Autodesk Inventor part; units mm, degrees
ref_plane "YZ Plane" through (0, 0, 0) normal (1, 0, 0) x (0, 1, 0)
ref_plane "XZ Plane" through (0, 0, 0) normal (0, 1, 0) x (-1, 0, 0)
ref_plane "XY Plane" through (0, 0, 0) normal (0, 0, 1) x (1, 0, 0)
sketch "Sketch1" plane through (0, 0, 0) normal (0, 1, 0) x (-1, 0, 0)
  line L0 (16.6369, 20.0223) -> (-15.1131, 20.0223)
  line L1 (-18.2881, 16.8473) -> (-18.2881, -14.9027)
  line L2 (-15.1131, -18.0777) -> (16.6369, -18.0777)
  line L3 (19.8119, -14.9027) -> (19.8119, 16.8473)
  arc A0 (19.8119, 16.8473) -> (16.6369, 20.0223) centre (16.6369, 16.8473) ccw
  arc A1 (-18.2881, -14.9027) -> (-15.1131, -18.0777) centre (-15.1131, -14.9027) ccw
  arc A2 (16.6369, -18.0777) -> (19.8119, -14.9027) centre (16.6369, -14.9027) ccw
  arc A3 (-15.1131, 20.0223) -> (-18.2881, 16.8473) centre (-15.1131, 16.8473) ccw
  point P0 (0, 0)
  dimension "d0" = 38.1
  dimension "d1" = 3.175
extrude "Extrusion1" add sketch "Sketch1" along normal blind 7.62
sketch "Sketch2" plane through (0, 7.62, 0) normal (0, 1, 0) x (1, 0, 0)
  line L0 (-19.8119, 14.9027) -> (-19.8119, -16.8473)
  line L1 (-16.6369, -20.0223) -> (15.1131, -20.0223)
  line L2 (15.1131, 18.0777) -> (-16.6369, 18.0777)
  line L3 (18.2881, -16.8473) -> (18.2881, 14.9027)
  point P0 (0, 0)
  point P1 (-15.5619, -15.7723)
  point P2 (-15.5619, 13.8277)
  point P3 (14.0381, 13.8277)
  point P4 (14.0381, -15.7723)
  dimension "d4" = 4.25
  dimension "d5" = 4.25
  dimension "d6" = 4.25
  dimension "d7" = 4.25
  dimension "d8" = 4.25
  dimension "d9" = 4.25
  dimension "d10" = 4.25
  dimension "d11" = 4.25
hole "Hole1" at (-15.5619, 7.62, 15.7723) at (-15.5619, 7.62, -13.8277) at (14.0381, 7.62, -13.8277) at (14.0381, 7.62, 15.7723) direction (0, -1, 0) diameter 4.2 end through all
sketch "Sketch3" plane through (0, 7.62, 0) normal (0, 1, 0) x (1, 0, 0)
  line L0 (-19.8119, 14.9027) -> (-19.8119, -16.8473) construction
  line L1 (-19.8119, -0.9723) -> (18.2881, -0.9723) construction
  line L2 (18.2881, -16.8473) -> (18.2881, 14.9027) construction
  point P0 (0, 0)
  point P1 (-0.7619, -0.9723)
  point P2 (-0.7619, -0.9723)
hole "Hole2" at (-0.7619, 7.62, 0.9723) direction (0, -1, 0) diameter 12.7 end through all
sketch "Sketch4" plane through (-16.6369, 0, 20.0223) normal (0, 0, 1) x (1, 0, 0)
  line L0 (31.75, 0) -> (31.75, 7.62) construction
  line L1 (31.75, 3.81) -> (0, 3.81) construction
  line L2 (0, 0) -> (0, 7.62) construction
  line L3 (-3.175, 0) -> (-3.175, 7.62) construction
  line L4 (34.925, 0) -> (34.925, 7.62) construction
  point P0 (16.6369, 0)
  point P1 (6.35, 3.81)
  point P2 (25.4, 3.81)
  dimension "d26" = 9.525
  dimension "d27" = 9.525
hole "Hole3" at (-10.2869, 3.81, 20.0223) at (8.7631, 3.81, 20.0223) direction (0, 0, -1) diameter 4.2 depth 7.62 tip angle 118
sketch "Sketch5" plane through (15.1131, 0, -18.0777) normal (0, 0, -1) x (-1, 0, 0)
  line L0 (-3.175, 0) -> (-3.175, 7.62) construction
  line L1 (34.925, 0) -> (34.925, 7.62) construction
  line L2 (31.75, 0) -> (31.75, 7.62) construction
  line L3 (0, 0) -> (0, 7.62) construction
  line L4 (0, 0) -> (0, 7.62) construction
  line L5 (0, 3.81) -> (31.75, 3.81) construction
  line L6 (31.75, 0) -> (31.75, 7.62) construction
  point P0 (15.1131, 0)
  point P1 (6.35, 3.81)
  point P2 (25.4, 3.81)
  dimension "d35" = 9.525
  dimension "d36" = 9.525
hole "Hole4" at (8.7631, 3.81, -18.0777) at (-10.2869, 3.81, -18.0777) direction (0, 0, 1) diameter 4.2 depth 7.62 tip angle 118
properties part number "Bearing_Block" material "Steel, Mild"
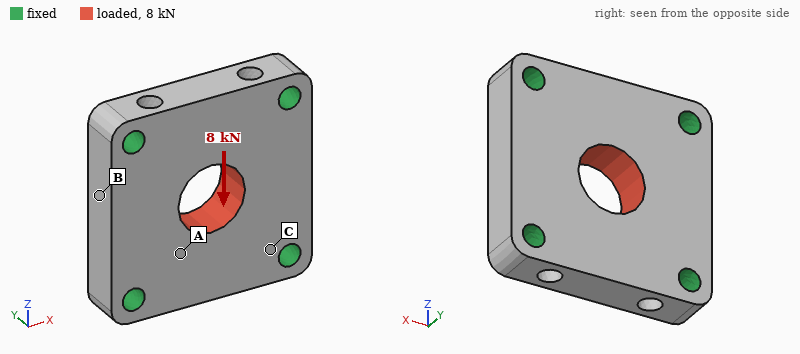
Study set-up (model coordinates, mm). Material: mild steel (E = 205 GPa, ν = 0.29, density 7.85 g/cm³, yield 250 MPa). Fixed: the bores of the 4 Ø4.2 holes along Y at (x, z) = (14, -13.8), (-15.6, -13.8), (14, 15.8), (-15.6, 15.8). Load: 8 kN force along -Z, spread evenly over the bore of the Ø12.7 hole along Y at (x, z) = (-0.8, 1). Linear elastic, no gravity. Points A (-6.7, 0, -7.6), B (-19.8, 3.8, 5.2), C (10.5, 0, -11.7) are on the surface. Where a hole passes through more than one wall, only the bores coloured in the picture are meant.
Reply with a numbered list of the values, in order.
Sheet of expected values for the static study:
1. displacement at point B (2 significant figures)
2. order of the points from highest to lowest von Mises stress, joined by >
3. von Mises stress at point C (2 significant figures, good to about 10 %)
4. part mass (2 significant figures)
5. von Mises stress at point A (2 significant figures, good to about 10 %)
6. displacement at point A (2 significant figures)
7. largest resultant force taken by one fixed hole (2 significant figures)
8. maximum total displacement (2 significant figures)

1. 0.55 µm
2. C > A > B
3. 43 MPa
4. 72 g
5. 26 MPa
6. 2.2 µm
7. 2.2 kN
8. 3.3 µm
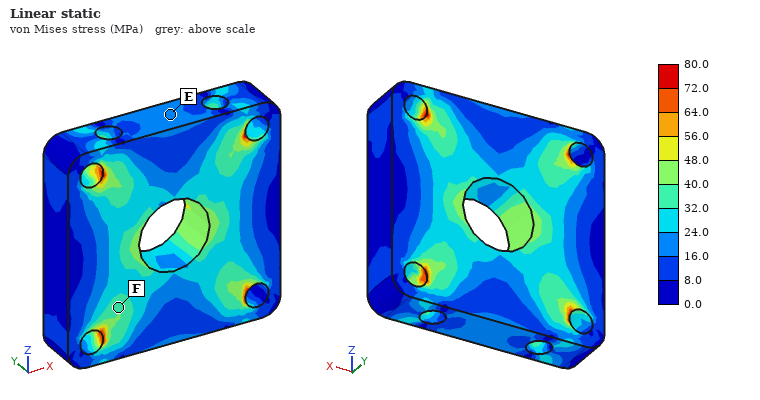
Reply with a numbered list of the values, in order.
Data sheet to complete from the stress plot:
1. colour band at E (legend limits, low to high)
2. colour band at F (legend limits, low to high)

1. 16.0 to 24.0 MPa
2. 32.0 to 40.0 MPa
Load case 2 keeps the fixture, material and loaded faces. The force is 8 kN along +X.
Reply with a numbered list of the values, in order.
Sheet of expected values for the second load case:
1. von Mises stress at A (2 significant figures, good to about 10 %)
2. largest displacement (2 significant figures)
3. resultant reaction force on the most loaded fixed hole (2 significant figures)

1. 28 MPa
2. 3.3 µm
3. 2.2 kN
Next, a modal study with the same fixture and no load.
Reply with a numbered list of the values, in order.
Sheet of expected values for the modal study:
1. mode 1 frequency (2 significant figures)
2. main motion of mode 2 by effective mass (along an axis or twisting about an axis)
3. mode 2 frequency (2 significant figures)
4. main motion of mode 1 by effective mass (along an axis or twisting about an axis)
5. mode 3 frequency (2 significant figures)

1. 25 kHz
2. twisting about X
3. 30 kHz
4. along Y
5. 35 kHz
